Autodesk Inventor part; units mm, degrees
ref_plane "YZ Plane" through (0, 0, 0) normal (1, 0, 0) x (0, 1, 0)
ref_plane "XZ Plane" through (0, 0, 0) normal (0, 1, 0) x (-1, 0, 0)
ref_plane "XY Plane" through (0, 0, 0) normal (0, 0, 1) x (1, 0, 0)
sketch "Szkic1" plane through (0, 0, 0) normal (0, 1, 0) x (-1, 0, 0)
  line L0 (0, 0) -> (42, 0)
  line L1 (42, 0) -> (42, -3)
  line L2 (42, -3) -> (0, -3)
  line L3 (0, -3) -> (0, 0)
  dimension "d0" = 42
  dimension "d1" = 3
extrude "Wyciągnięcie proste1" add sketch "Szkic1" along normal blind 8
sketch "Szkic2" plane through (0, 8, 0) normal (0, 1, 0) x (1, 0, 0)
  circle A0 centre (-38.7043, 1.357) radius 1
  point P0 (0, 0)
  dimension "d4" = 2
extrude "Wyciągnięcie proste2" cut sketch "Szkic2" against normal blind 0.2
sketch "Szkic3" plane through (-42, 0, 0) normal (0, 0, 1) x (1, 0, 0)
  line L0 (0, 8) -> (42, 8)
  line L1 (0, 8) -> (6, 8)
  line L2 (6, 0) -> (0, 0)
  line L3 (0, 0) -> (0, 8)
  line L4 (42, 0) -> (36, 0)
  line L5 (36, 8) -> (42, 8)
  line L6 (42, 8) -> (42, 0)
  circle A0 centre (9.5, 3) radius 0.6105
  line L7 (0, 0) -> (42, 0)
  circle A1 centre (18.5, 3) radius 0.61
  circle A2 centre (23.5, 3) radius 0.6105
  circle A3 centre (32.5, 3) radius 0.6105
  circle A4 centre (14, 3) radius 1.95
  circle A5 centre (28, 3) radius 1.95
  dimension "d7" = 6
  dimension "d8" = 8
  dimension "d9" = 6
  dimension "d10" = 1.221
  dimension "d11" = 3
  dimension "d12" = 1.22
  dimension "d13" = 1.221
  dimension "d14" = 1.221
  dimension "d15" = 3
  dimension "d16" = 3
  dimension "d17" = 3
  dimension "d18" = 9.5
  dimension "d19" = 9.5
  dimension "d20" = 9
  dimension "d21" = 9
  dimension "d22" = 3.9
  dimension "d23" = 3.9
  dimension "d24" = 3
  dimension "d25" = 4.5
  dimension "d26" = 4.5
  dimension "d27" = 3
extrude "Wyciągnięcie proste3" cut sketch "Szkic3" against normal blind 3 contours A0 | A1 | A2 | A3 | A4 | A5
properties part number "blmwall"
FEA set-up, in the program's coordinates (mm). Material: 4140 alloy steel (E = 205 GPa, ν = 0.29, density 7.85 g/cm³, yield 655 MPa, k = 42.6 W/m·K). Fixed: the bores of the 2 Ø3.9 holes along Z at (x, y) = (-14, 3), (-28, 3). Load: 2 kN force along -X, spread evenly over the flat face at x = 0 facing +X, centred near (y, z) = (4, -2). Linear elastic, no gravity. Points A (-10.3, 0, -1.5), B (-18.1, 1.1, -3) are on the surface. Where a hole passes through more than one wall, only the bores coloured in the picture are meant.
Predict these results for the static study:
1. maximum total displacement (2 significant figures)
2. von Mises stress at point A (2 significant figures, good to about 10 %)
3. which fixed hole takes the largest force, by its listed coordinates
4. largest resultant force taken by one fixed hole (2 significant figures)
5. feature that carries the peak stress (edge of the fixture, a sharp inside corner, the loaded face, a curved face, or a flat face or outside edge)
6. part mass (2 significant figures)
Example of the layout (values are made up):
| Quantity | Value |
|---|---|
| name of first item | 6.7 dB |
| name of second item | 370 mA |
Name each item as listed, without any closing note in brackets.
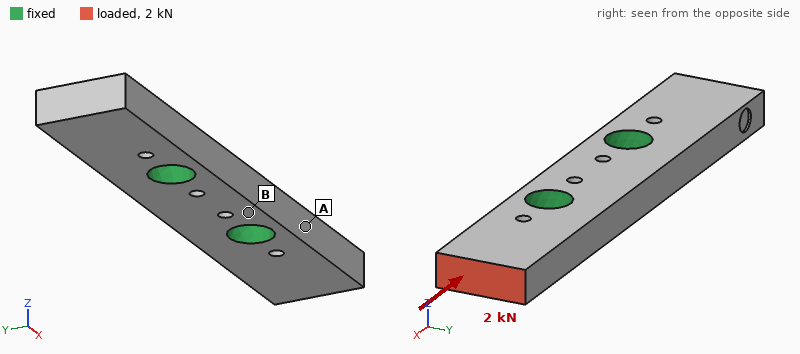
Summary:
| Quantity | Value |
|---|---|
| maximum total displacement | 7.1 µm |
| von Mises stress at point A | 57 MPa |
| which fixed hole takes the largest force, by its listed coordinates | (-14, 3) |
| largest resultant force taken by one fixed hole | 1.9 kN |
| feature that carries the peak stress | a curved face |
| part mass | 7.2 g |
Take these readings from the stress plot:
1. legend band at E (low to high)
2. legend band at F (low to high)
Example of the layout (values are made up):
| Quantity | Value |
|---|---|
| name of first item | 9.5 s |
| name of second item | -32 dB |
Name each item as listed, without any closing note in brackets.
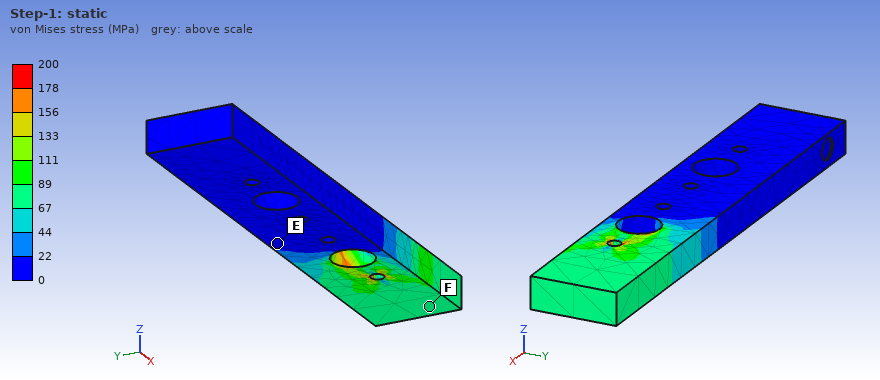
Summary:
| Quantity | Value |
|---|---|
| legend band at E | 0 to 22 MPa |
| legend band at F | 67 to 89 MPa |
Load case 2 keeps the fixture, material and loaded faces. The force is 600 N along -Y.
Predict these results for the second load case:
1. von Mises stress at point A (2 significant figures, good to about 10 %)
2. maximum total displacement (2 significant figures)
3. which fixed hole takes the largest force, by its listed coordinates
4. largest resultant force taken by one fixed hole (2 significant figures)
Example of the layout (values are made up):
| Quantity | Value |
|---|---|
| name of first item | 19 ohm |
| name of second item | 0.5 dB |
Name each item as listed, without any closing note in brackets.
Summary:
| Quantity | Value |
|---|---|
| von Mises stress at point A | 220 MPa |
| maximum total displacement | 30 µm |
| which fixed hole takes the largest force, by its listed coordinates | (-14, 3) |
| largest resultant force taken by one fixed hole | 760 N |
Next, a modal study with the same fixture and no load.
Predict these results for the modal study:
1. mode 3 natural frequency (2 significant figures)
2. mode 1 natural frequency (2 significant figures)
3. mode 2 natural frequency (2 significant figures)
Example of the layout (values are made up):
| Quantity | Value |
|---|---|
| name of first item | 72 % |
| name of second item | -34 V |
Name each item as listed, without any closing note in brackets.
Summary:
| Quantity | Value |
|---|---|
| mode 3 natural frequency | 27 kHz |
| mode 1 natural frequency | 14 kHz |
| mode 2 natural frequency | 14 kHz |
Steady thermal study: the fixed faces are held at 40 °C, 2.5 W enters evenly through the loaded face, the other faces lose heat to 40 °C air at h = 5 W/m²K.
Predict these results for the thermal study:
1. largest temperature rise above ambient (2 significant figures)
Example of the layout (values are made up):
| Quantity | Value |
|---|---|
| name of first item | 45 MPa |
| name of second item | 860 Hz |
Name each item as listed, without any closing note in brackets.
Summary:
| Quantity | Value |
|---|---|
| largest temperature rise above ambient | 32 K |
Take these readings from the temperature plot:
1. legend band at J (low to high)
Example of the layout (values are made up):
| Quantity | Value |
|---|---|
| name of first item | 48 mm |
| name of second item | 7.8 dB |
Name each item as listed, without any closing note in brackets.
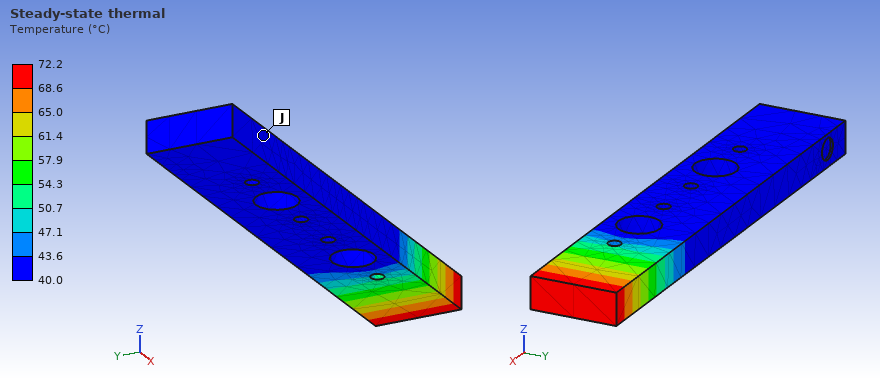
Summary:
| Quantity | Value |
|---|---|
| legend band at J | 40.0 to 43.6 °C |
